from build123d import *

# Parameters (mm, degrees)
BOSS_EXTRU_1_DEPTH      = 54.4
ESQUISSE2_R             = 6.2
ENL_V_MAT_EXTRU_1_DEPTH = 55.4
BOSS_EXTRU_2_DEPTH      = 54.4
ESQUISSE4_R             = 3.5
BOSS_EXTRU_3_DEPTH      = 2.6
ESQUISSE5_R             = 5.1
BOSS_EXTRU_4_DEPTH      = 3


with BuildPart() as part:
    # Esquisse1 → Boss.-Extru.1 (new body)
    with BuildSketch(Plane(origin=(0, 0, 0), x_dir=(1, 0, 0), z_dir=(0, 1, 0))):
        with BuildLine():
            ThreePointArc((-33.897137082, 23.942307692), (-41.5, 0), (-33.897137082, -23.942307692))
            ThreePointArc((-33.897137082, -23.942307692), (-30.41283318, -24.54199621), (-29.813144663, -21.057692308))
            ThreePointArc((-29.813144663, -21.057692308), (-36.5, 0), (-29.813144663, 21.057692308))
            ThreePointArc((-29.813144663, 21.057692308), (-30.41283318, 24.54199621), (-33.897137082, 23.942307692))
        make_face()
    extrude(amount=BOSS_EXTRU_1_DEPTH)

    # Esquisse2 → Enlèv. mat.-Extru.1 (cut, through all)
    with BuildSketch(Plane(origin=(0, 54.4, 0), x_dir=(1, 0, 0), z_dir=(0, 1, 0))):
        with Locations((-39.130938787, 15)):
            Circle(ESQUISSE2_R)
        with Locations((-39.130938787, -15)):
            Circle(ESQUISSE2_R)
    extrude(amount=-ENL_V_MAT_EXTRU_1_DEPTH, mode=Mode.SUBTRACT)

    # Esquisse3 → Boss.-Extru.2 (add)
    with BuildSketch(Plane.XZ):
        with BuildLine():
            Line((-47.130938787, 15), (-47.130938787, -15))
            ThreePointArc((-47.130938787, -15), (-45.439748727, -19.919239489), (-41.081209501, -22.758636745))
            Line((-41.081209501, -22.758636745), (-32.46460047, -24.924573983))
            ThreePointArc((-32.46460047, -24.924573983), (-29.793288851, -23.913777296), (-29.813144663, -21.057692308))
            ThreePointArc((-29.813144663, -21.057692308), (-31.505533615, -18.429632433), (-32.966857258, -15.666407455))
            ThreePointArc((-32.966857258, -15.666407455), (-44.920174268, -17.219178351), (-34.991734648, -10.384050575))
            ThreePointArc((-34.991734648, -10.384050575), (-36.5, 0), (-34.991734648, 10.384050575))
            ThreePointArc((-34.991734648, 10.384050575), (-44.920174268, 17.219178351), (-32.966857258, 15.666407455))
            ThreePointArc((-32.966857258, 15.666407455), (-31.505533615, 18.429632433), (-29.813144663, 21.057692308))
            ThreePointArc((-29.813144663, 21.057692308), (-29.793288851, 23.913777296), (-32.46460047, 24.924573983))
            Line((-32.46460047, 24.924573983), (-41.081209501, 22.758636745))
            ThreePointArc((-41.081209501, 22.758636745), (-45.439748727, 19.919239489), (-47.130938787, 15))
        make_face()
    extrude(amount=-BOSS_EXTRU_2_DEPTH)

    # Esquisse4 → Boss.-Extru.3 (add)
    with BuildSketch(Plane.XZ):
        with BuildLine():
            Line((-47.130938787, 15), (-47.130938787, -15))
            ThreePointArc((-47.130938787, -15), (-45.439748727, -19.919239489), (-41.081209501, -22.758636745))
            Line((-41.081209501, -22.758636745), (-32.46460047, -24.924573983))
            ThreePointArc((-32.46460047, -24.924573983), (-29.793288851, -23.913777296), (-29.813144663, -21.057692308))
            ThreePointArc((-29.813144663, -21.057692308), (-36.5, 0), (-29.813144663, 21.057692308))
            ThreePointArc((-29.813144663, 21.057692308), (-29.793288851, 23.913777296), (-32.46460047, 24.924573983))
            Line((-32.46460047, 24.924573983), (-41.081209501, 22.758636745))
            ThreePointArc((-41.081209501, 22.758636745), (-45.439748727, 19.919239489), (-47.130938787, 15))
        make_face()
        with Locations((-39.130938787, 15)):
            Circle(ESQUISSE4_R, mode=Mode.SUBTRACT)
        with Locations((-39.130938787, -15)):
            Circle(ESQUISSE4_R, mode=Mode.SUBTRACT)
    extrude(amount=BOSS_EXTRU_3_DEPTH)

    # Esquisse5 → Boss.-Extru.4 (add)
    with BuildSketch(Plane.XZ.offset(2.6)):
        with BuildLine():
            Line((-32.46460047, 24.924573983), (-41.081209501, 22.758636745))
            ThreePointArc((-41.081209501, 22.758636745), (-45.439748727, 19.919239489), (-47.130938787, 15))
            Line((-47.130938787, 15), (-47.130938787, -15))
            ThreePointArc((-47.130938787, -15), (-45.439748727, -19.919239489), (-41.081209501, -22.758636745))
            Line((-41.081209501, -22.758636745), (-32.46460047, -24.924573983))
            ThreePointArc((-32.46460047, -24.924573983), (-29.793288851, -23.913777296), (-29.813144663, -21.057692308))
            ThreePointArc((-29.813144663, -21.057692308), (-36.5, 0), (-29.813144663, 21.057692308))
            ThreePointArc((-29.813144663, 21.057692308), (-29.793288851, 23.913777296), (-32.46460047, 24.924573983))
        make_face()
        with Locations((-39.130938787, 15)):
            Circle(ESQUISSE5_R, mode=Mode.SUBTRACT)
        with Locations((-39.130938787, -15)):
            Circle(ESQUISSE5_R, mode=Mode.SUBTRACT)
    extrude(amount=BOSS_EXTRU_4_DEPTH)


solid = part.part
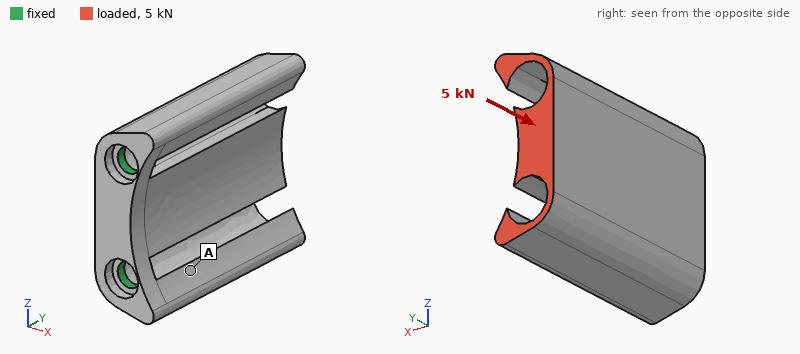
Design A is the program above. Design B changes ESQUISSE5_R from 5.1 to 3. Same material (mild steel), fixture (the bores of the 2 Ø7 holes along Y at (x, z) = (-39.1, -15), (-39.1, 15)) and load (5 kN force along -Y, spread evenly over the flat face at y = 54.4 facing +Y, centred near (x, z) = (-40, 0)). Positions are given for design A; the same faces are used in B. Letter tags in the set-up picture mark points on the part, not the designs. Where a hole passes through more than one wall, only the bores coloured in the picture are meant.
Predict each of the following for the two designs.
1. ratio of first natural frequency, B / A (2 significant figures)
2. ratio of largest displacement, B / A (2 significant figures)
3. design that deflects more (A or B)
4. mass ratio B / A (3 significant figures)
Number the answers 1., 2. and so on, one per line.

1. 1.2
2. 0.86
3. A
4. 1.01
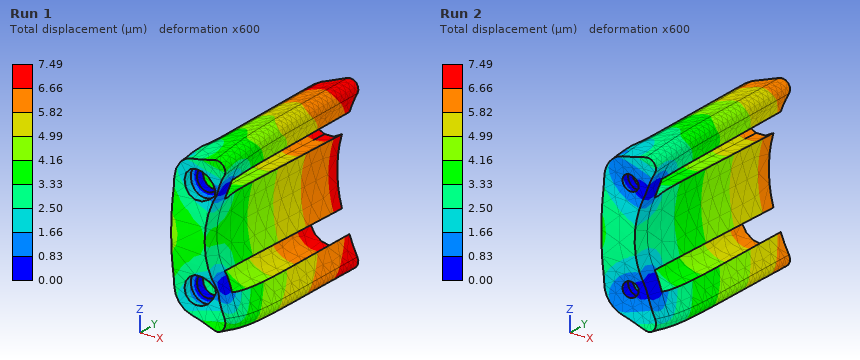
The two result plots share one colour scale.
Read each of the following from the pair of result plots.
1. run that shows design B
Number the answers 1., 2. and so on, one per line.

1. Run 2
